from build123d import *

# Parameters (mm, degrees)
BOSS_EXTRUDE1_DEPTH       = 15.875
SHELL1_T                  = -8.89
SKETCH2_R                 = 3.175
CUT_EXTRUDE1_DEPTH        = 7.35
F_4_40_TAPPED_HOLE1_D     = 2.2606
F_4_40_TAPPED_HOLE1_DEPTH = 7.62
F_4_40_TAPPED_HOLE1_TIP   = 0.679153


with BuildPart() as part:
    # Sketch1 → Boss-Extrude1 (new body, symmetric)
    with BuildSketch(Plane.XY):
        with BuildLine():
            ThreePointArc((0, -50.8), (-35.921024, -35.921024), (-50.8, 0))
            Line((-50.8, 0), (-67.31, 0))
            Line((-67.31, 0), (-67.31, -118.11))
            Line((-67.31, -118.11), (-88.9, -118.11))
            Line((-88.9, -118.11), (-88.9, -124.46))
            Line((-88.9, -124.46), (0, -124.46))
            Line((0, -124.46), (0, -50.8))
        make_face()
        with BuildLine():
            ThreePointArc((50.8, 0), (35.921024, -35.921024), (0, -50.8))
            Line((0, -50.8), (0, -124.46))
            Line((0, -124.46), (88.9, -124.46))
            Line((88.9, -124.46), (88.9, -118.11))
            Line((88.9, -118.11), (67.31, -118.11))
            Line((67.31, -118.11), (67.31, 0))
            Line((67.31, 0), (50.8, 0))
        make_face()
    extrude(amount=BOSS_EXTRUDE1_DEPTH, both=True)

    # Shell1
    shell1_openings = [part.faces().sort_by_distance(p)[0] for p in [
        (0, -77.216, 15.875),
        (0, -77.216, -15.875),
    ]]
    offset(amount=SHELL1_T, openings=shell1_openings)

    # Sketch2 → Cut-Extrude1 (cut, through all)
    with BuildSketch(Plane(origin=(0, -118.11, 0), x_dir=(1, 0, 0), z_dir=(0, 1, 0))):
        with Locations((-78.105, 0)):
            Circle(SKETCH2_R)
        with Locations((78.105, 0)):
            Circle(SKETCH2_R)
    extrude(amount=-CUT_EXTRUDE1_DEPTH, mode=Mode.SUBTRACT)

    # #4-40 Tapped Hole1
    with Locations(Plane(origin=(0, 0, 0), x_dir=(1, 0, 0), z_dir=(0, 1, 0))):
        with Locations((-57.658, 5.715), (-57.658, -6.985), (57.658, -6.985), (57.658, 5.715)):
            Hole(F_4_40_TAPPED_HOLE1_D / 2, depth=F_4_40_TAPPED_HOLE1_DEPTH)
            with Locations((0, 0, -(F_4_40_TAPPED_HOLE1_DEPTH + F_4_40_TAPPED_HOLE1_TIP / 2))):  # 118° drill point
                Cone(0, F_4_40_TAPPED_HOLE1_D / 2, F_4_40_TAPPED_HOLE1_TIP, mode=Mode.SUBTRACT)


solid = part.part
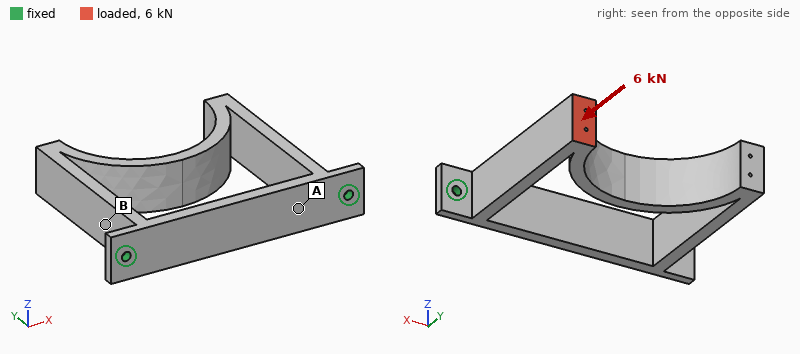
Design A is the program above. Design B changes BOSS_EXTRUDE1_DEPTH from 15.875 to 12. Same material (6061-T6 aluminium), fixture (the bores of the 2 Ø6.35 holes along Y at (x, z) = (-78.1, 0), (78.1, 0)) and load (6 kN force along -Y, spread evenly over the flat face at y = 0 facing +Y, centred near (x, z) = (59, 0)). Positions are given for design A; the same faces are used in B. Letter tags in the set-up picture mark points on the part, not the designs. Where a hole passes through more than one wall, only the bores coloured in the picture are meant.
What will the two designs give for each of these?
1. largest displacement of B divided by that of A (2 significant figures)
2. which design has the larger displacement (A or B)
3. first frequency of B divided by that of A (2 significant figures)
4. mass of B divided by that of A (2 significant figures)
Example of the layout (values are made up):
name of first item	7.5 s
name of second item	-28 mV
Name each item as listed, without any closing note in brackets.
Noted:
largest displacement of B divided by that of A	1.3
which design has the larger displacement	B
first frequency of B divided by that of A	0.98
mass of B divided by that of A	0.76
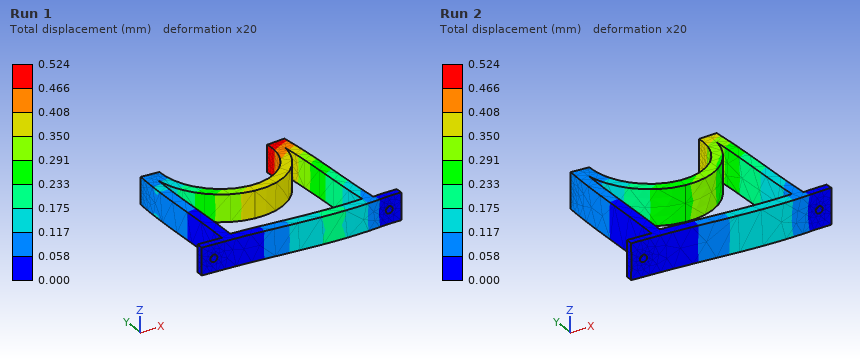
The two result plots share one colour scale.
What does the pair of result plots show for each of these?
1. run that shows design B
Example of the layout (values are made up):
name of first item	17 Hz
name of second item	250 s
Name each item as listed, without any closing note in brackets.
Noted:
run that shows design B	Run 1
